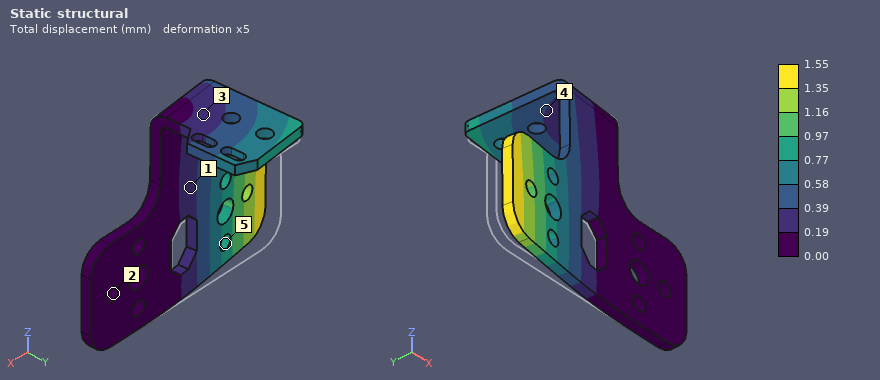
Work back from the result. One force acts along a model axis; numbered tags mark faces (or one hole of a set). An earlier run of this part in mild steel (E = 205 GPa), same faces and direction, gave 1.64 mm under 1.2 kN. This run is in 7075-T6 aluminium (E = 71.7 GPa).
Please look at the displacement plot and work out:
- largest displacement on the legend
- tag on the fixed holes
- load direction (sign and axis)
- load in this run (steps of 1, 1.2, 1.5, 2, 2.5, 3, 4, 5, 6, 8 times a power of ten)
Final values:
1.55 mm
2
-Y
400 N
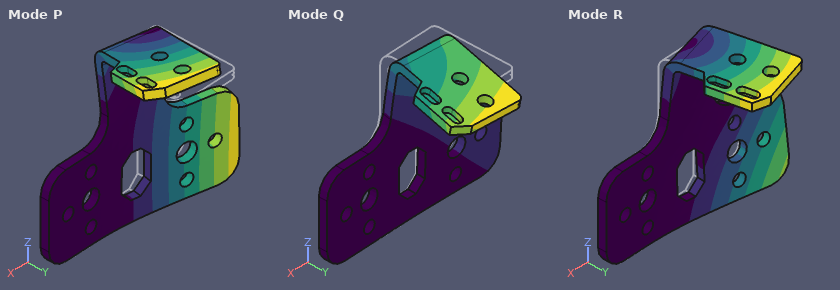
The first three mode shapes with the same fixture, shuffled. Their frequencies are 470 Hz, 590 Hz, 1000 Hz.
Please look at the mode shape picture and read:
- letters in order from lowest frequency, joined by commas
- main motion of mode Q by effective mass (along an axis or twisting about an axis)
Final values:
Q, P, R
along Y
